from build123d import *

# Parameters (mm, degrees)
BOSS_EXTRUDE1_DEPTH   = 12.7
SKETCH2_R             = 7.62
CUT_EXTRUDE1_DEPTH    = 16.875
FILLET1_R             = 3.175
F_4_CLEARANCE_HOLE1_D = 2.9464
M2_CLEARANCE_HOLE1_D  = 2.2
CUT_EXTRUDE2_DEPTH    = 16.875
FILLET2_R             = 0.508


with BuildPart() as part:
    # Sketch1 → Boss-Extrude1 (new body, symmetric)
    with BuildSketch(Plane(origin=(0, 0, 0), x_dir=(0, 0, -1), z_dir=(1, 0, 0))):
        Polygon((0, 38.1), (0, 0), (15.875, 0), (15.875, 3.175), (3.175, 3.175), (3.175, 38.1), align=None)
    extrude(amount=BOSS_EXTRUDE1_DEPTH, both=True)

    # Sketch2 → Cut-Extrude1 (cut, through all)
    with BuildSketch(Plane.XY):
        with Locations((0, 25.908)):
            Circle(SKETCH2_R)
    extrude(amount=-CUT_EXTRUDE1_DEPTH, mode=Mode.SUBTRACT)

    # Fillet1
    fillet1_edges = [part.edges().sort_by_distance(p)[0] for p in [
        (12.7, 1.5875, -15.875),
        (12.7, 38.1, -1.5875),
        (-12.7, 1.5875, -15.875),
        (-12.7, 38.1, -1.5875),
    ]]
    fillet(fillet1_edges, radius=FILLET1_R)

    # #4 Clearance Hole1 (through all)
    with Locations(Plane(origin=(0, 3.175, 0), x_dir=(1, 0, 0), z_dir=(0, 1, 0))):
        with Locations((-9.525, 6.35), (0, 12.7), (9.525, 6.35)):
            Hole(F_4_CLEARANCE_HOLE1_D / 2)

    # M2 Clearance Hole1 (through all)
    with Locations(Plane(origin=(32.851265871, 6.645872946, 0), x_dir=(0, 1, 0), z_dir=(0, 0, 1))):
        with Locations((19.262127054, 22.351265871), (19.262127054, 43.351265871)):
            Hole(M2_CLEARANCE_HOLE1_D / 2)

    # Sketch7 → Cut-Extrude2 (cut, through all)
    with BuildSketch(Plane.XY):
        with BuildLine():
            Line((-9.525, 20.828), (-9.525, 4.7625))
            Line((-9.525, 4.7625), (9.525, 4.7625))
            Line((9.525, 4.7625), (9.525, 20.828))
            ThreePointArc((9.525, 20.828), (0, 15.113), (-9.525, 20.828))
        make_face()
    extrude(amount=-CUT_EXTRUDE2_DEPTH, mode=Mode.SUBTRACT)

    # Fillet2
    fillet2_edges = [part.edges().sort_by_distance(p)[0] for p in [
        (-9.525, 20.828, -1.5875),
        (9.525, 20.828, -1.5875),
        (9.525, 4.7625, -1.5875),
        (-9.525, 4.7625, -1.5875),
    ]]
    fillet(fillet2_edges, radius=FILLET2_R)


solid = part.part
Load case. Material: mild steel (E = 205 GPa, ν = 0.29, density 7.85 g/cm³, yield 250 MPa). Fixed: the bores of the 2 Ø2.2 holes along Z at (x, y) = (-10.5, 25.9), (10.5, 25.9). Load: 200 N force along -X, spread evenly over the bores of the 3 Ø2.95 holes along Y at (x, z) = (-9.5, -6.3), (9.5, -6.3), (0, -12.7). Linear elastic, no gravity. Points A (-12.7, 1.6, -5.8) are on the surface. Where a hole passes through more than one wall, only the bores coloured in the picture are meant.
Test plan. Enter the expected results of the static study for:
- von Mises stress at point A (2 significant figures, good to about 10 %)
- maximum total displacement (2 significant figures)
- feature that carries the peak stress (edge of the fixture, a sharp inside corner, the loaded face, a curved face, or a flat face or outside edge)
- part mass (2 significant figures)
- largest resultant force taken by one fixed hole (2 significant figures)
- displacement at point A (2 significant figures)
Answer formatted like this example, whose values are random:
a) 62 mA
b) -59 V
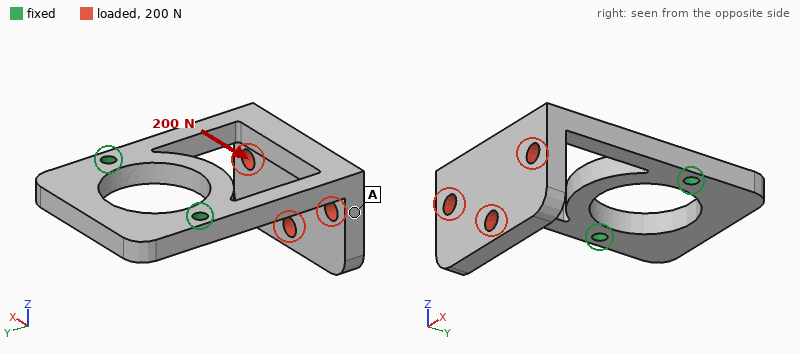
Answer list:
a) 24 MPa
b) 83 µm
c) a curved face
d) 21 g
e) 180 N
f) 62 µm
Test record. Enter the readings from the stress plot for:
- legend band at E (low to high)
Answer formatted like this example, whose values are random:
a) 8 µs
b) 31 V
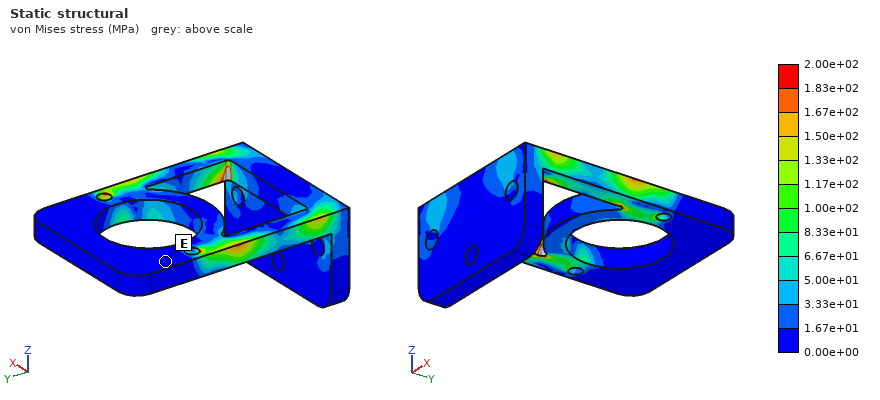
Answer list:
a) 0.00e+00 to 1.67e+01 MPa
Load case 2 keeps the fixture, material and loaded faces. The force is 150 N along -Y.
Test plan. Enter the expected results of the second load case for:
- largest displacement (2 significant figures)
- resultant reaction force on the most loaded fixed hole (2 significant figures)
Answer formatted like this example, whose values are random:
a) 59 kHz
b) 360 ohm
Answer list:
a) 0.13 mm
b) 75 N
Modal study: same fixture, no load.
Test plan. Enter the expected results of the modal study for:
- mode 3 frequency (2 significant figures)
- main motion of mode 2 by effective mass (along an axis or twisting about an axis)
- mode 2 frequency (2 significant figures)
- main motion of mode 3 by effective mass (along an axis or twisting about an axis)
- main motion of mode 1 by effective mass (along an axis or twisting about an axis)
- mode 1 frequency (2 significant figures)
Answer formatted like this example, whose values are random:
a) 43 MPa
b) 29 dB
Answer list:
a) 4600 Hz
b) along X
c) 2700 Hz
d) along X
e) along Z
f) 1300 Hz
